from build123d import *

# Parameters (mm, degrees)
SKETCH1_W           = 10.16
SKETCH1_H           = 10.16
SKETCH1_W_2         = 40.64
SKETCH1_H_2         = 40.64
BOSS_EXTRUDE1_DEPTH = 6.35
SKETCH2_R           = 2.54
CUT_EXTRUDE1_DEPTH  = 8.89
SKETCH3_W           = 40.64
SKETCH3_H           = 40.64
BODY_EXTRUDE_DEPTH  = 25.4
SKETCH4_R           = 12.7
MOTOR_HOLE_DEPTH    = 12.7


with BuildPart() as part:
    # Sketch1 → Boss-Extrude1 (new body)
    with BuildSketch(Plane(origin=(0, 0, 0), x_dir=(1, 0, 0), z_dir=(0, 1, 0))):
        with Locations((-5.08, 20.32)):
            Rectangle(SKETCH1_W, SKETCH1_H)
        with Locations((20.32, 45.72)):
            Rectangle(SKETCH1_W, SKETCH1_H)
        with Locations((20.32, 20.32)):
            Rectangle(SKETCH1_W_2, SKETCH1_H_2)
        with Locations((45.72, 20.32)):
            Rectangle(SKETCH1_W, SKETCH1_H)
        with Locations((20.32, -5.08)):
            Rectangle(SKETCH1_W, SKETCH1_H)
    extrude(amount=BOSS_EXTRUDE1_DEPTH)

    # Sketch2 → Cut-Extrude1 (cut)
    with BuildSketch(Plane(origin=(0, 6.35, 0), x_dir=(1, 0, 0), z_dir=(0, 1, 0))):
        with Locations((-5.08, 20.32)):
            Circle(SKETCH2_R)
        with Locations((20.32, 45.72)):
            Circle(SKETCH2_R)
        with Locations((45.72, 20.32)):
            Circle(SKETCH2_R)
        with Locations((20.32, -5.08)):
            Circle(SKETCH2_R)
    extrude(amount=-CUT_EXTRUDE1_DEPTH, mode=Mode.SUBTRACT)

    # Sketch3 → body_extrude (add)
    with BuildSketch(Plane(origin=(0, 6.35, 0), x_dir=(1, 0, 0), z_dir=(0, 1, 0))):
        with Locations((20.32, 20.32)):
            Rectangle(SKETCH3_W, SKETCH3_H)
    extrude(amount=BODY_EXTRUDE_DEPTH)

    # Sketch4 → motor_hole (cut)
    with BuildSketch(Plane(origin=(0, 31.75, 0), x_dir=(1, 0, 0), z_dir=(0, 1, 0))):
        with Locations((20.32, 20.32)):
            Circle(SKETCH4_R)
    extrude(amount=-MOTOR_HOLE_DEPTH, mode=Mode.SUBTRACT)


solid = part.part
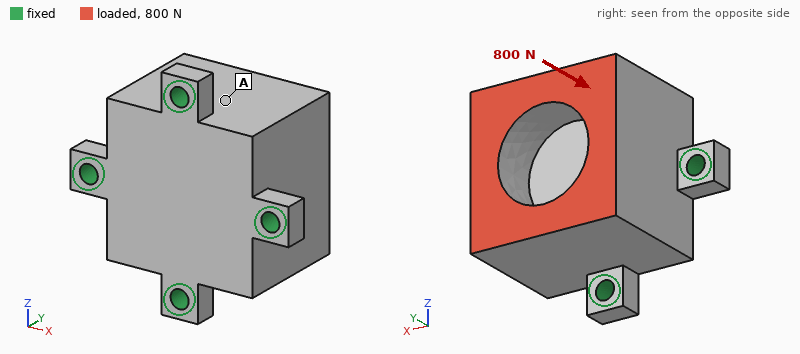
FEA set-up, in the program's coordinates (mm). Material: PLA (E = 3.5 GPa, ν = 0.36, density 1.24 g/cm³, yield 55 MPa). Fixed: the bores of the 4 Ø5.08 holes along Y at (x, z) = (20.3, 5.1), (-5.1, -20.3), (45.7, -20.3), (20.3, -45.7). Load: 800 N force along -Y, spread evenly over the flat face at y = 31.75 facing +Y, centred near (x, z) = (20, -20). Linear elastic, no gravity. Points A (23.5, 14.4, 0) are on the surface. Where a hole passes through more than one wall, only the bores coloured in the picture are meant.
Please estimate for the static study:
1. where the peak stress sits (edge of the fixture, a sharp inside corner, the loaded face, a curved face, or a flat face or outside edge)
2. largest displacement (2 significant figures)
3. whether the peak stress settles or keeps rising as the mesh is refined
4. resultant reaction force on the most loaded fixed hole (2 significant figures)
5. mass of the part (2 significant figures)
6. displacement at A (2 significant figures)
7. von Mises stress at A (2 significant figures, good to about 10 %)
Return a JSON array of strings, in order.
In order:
["edge of the fixture", "27 µm", "keeps rising", "210 N", "60 g", "22 µm", "1.3 MPa"]
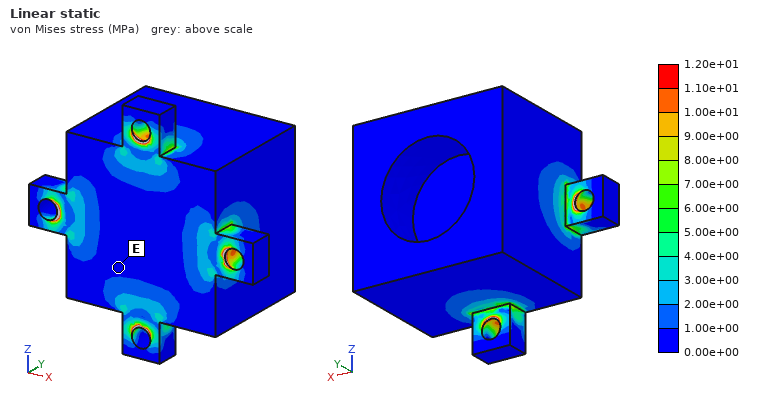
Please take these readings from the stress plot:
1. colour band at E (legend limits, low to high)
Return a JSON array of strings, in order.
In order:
["0.00e+00 to 1.00e+00 MPa"]
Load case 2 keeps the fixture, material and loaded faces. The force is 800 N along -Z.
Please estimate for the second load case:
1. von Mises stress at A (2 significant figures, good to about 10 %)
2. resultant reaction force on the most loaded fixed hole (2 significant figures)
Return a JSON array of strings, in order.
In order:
["3.5 MPa", "610 N"]
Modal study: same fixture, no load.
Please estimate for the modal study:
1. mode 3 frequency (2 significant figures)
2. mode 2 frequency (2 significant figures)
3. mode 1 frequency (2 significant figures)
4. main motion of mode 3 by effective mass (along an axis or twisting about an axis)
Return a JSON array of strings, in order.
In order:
["4000 Hz", "3100 Hz", "3100 Hz", "along Y"]
